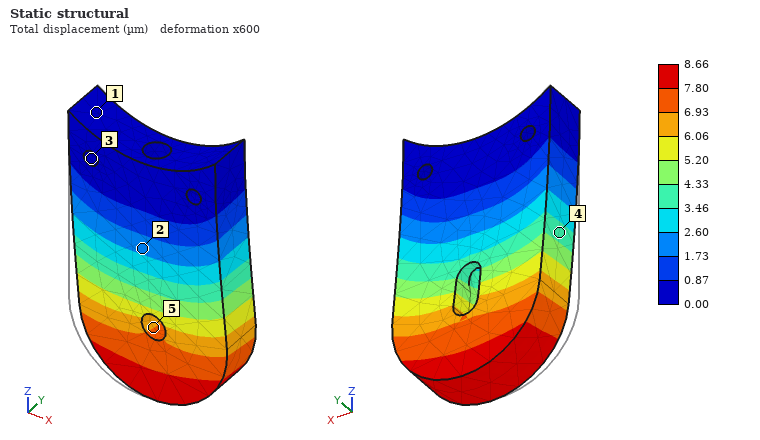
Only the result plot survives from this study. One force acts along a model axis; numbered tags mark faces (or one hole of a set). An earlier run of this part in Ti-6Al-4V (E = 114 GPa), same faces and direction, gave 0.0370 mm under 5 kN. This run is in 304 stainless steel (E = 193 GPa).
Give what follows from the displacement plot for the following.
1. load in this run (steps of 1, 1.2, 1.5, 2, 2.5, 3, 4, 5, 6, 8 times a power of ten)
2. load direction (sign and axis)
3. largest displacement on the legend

2 kN
+X
8.66 µm
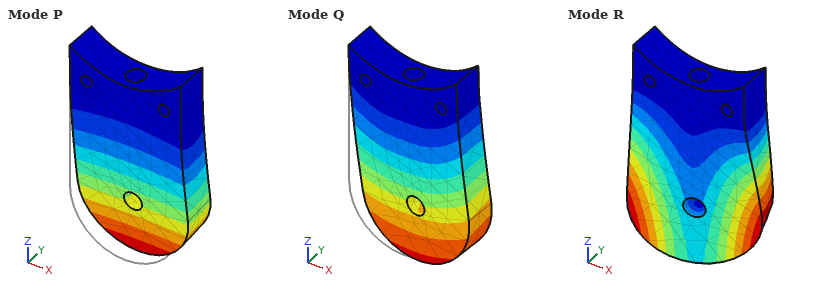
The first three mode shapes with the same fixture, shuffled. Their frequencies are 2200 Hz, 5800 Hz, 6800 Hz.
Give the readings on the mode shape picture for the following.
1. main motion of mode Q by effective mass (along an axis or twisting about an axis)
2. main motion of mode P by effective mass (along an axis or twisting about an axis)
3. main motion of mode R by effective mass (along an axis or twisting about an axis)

along X
along Y
twisting about Z
